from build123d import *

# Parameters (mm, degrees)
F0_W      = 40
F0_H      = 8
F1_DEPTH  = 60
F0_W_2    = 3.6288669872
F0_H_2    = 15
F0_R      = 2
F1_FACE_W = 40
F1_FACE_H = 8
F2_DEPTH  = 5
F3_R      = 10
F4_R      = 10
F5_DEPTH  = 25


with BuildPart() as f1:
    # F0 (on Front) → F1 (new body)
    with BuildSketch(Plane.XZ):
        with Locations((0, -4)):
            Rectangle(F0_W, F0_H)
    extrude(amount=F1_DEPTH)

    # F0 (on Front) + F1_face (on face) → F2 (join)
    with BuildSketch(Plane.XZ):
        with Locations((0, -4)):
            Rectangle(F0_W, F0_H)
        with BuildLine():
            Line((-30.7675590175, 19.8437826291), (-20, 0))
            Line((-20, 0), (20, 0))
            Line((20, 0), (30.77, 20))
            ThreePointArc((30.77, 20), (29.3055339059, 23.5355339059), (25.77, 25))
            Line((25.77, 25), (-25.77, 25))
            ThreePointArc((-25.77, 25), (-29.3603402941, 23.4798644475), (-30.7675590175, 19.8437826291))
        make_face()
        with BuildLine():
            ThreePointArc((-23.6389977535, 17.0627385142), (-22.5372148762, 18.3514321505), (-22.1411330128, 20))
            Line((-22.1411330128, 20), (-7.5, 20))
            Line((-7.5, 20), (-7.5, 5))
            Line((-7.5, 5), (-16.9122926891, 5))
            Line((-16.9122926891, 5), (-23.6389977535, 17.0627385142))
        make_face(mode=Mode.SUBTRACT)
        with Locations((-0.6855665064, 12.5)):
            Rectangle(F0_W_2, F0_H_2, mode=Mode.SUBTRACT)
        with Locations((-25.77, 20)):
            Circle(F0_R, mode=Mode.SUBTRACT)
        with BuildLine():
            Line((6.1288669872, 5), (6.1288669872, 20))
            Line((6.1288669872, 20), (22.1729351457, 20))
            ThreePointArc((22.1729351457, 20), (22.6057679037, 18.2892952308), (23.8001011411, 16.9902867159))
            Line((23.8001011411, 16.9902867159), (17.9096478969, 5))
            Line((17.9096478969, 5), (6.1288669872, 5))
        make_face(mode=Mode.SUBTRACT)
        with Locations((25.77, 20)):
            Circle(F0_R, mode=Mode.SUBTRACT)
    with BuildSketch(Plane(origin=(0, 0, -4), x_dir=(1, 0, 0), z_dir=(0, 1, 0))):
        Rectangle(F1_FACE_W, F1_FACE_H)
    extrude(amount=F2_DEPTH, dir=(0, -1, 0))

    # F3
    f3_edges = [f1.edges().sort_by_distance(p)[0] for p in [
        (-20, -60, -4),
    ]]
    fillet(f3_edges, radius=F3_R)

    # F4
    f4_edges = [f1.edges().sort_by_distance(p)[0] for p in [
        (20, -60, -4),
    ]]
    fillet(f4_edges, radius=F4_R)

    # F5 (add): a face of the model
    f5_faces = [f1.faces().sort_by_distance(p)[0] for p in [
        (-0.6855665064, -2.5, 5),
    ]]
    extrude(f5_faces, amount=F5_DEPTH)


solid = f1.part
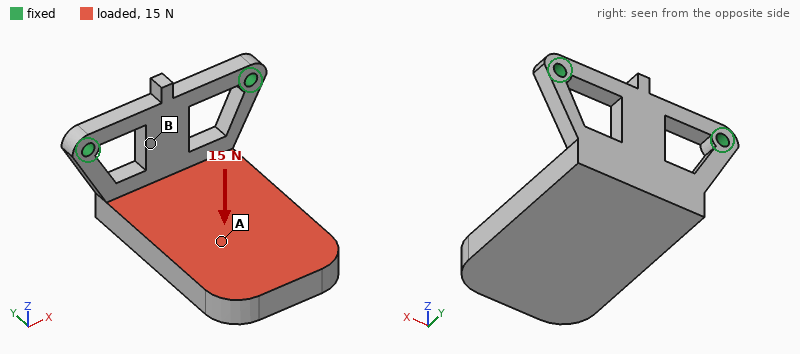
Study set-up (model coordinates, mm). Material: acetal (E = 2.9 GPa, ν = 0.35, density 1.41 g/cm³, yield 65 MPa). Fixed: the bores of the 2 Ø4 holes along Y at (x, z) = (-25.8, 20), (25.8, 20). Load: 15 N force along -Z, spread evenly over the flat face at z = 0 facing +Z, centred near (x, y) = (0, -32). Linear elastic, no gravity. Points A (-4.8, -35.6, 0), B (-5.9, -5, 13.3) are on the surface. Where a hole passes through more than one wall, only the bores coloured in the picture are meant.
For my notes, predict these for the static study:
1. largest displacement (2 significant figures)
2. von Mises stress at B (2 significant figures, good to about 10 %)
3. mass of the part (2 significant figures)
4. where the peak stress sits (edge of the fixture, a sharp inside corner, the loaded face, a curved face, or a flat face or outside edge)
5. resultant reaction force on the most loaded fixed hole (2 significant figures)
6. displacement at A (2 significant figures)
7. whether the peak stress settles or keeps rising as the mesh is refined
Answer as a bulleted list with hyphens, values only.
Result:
- 1.1 mm
- 3.1 MPa
- 33 g
- edge of the fixture
- 8.4 N
- 0.61 mm
- keeps rising
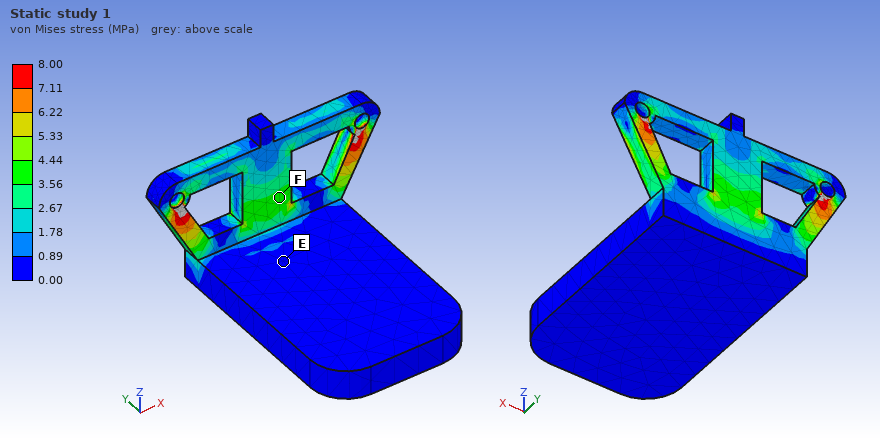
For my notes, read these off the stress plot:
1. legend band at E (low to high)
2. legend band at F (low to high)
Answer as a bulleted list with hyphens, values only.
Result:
- 0.00 to 0.89 MPa
- 3.56 to 4.44 MPa
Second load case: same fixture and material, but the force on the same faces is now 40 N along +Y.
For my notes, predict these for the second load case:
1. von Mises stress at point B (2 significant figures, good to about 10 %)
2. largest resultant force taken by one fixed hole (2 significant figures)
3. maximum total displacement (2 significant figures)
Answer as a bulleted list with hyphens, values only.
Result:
- 2.2 MPa
- 20 N
- 1.0 mm
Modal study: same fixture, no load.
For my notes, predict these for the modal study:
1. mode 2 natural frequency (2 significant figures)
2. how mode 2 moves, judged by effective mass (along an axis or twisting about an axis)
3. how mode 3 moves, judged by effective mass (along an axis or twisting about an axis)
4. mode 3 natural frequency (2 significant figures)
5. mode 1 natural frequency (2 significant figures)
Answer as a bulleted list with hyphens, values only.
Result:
- 360 Hz
- along X
- along Y
- 610 Hz
- 140 Hz
